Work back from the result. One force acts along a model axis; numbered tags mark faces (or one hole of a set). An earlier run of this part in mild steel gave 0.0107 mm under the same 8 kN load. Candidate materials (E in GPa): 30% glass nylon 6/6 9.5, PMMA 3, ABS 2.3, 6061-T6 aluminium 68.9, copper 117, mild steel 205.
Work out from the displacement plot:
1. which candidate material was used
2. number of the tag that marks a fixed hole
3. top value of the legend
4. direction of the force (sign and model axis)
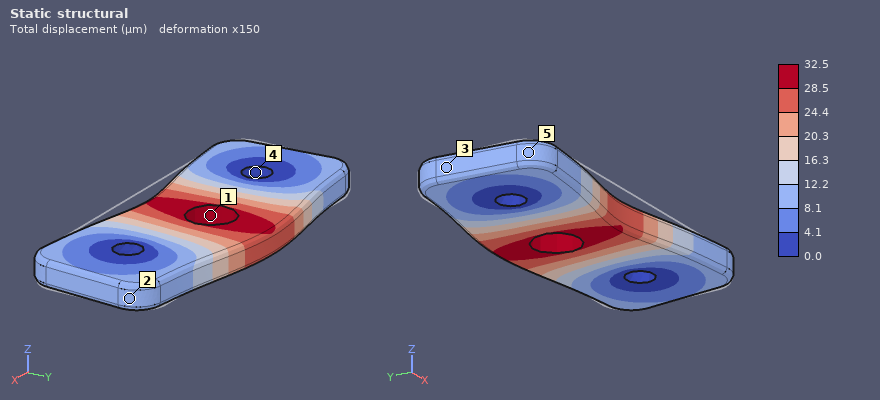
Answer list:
6061-T6 aluminium
4
32.5 µm
+Y
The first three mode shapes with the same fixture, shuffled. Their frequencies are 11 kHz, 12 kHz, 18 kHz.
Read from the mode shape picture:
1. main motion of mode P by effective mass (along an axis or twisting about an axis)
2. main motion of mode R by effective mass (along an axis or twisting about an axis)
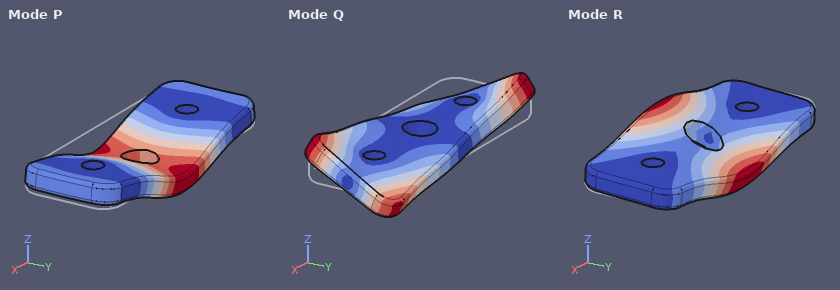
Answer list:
along Z
twisting about X
